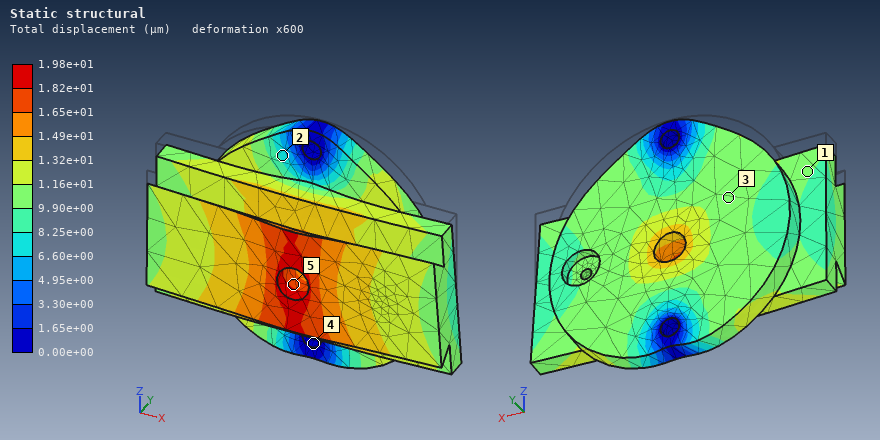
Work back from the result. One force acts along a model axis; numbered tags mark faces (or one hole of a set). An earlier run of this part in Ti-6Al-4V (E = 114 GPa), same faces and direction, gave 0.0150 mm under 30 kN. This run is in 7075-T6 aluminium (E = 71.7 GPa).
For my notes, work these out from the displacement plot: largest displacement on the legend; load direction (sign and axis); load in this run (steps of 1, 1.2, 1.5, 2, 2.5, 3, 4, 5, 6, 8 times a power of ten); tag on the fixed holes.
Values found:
1.98e+01 µm
-Z
25 kN
4
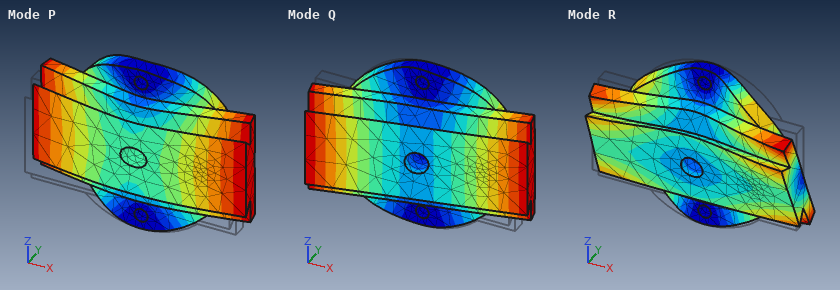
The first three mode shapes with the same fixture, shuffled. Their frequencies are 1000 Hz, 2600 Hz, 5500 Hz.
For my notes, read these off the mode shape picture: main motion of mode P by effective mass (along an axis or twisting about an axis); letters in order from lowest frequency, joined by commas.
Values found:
along Y
Q, P, R
